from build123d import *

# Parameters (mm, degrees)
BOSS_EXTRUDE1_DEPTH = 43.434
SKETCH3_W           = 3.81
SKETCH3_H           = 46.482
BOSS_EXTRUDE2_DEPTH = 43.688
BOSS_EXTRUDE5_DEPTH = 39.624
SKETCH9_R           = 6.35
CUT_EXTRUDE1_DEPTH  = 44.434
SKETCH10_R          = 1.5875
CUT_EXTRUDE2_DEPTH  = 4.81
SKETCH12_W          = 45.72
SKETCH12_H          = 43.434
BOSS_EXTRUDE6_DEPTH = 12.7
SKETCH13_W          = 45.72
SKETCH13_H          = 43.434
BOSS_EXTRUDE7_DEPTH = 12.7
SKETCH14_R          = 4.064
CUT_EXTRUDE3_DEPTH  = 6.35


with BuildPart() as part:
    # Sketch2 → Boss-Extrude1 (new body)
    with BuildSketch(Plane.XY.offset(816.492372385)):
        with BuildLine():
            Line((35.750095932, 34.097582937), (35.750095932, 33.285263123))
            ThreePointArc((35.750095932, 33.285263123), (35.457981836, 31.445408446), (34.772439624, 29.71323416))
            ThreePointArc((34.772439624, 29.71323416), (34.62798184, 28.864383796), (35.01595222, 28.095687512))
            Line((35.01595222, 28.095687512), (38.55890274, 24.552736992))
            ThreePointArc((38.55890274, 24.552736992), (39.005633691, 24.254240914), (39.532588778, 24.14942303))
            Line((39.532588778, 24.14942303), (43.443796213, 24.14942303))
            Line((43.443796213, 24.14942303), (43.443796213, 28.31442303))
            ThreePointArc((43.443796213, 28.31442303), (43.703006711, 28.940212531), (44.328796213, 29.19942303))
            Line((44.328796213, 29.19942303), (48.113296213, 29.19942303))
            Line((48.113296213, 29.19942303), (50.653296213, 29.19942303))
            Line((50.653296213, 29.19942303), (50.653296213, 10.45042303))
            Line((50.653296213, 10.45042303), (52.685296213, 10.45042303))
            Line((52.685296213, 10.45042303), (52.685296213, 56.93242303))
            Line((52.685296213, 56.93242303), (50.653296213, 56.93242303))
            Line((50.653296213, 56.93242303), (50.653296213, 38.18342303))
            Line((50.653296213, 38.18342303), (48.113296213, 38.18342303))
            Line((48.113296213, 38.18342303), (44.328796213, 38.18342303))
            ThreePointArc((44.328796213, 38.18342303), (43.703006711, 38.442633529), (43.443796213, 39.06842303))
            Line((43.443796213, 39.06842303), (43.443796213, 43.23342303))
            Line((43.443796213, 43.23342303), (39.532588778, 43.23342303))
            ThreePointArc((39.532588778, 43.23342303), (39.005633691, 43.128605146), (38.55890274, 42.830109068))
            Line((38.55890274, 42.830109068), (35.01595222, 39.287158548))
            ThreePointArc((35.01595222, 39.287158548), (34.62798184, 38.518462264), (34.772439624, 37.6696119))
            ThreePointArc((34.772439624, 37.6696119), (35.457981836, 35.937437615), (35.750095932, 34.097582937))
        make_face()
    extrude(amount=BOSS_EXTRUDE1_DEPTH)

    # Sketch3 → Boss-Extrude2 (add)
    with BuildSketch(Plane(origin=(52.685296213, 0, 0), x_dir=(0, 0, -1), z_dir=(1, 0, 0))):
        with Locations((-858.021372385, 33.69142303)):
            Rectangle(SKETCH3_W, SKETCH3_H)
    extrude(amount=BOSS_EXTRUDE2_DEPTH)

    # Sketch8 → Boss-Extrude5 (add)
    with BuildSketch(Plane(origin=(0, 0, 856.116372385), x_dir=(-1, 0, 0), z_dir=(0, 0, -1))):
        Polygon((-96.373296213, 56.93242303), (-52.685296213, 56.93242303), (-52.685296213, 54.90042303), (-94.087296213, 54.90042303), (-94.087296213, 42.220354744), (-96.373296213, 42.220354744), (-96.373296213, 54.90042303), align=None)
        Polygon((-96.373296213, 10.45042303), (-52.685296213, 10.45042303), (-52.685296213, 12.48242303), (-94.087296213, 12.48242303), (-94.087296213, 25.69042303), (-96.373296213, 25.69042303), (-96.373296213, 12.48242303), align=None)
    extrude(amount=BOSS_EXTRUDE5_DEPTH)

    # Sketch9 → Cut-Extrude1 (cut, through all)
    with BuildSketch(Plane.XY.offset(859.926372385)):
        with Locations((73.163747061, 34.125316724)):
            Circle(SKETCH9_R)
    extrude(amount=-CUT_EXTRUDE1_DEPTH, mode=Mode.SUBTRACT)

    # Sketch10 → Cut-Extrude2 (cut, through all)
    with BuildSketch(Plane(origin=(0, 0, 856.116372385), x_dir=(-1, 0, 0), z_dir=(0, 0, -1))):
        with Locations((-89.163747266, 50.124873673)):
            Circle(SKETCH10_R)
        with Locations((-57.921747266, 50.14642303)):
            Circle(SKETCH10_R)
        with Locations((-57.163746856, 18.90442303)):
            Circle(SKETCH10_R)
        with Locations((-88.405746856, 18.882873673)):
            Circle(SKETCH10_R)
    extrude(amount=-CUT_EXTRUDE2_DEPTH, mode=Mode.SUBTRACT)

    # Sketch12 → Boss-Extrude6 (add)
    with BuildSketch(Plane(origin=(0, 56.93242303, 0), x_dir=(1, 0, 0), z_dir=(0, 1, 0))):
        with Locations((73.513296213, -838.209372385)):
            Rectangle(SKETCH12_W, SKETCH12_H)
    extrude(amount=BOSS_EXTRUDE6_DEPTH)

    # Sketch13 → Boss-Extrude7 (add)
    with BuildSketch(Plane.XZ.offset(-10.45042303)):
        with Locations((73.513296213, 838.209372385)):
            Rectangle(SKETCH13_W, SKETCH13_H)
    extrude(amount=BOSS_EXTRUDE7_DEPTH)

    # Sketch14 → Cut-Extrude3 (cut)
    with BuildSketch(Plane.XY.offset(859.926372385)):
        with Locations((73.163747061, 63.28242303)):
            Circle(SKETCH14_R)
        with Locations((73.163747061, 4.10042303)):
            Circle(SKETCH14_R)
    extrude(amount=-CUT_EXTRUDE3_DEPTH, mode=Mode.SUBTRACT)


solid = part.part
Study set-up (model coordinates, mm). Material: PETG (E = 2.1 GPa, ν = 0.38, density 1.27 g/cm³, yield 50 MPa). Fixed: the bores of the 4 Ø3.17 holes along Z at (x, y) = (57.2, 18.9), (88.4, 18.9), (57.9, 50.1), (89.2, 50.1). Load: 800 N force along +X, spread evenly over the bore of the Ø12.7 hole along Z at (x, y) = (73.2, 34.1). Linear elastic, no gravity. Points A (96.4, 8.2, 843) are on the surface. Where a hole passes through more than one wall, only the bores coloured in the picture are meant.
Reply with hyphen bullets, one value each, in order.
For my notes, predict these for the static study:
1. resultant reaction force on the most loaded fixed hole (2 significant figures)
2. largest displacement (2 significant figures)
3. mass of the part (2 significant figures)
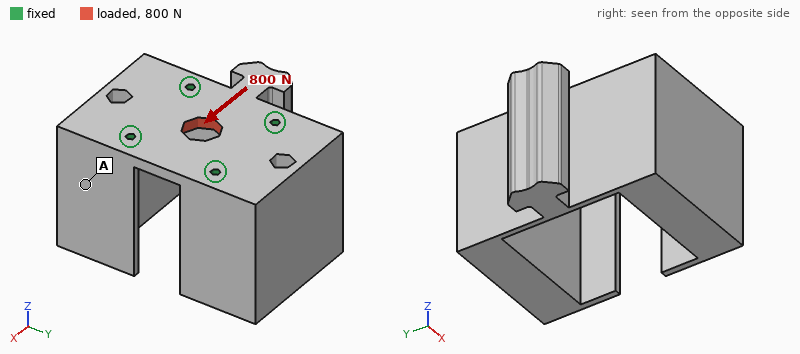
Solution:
- 220 N
- 57 µm
- 100 g
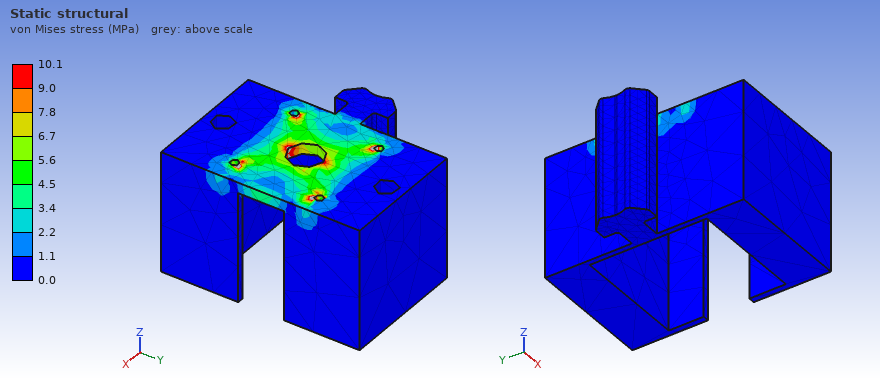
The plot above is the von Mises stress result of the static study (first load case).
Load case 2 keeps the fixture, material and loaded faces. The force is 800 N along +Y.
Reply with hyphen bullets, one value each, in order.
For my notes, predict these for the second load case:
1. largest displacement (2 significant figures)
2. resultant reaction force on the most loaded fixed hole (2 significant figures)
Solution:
- 46 µm
- 210 N
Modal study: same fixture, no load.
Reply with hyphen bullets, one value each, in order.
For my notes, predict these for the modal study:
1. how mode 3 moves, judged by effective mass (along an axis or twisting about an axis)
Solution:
- along Z
